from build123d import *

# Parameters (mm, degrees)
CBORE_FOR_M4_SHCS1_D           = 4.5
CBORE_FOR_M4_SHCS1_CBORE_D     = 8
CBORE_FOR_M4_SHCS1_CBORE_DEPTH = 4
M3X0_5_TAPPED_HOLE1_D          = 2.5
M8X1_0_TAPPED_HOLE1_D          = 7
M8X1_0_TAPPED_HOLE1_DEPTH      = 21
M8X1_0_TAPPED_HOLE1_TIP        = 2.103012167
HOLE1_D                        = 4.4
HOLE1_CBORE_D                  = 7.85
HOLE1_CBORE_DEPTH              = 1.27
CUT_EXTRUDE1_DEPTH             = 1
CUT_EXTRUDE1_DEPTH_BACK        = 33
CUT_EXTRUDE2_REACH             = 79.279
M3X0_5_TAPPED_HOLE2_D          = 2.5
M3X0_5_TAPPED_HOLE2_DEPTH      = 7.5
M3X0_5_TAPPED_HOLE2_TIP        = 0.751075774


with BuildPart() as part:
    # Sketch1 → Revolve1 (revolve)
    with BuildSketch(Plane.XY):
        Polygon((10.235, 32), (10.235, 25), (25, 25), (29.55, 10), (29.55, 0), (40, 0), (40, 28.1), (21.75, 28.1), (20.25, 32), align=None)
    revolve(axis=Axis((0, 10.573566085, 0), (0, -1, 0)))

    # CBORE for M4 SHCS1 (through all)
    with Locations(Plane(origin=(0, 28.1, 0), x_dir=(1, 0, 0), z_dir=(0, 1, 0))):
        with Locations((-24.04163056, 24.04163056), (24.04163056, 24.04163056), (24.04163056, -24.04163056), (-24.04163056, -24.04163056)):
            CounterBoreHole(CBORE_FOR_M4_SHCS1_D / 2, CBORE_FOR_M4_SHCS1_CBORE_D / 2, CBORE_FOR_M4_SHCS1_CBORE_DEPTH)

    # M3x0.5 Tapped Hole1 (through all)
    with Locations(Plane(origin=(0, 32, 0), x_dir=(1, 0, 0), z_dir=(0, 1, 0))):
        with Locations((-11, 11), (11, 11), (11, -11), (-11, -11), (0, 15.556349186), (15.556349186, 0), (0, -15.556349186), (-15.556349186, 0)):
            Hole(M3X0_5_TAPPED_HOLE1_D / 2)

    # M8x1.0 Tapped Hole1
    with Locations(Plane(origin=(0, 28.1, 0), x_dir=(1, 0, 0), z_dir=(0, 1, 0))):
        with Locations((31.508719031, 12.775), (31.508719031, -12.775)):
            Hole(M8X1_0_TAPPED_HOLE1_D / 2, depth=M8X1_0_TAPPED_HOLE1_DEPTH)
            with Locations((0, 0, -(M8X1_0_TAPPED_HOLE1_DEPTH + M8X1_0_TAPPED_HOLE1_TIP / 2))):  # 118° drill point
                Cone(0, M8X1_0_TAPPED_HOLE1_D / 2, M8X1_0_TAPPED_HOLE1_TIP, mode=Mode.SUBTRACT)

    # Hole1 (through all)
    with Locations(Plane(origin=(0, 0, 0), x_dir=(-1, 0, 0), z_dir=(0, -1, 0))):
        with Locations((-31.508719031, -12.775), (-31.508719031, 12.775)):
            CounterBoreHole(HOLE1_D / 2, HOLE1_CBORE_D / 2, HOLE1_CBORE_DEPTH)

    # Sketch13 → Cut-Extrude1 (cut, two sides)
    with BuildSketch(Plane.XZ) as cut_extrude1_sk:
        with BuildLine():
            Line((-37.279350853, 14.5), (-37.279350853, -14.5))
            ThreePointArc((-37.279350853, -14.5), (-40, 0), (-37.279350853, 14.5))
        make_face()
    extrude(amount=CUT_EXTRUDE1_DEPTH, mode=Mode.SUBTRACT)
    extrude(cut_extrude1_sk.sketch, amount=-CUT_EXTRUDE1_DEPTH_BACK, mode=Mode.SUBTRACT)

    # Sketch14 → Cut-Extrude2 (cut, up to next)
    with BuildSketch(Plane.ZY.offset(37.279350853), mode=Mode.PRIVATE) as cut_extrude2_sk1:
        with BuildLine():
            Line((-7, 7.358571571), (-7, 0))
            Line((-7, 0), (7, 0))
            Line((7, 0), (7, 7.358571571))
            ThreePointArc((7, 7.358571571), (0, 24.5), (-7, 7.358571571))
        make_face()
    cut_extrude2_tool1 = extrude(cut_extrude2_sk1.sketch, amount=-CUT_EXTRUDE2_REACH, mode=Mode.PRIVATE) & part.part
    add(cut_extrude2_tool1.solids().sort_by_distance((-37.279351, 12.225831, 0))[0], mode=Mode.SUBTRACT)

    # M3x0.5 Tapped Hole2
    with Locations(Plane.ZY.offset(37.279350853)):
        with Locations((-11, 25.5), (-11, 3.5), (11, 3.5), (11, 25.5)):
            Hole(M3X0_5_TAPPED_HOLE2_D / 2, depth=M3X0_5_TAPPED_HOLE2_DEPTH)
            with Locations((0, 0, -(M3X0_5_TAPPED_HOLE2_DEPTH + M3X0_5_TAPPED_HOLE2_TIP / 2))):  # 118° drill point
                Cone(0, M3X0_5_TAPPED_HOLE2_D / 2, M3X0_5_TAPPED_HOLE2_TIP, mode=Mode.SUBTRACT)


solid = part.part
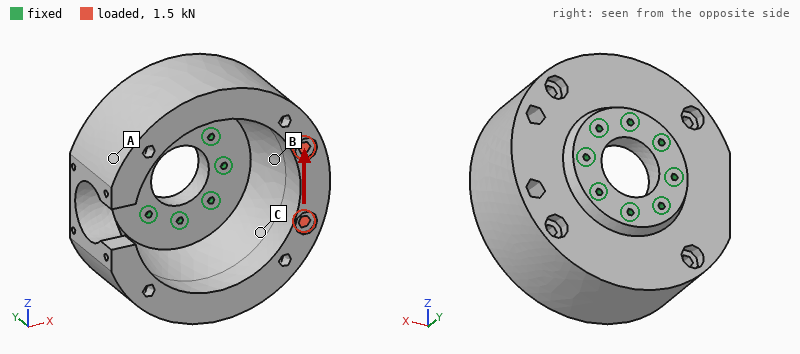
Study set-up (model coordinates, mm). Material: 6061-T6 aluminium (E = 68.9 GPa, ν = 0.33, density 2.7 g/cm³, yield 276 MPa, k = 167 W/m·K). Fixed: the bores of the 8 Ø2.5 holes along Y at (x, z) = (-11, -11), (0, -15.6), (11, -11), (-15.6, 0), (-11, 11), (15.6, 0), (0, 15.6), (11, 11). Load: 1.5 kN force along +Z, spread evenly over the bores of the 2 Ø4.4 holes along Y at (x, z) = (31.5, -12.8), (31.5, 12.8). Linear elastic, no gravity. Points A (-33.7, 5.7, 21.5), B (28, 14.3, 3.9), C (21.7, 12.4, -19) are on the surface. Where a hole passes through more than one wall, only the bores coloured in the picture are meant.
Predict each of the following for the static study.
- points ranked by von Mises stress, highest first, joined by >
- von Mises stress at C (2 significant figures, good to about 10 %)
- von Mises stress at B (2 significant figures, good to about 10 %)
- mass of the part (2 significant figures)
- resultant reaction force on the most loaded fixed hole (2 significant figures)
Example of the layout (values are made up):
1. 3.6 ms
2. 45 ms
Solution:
1. B > C > A
2. 7.4 MPa
3. 17 MPa
4. 190 g
5. 840 N
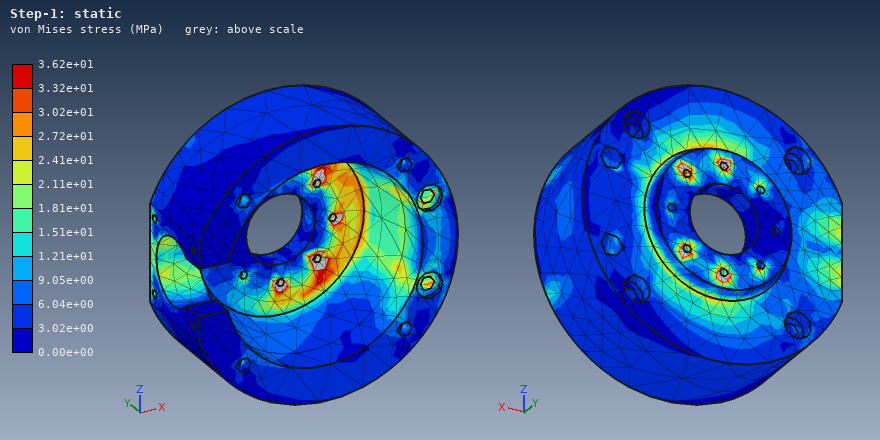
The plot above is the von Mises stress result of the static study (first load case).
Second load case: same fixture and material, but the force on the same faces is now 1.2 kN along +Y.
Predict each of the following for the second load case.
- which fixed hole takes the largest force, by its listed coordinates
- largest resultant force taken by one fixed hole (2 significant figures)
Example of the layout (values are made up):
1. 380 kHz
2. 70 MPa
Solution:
1. (15.6, 0)
2. 720 N
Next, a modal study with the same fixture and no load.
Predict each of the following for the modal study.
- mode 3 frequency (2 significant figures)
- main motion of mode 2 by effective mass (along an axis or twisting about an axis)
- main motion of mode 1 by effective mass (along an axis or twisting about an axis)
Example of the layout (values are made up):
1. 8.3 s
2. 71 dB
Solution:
1. 5100 Hz
2. along Z
3. along X
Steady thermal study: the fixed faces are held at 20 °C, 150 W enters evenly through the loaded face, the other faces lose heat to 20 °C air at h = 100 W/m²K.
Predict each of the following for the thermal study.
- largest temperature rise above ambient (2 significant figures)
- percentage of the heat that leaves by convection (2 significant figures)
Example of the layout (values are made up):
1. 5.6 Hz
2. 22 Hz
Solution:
1. 71 K
2. 28 %
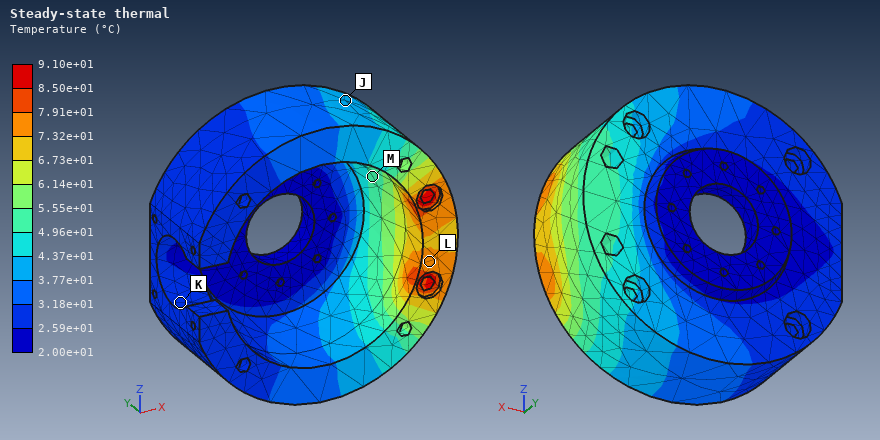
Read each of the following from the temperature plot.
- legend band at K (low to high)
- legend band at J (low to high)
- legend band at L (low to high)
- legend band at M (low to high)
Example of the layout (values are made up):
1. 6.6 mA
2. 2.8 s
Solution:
1. 2.59e+01 to 3.18e+01 °C
2. 3.77e+01 to 4.37e+01 °C
3. 7.32e+01 to 7.91e+01 °C
4. 4.96e+01 to 5.55e+01 °C
